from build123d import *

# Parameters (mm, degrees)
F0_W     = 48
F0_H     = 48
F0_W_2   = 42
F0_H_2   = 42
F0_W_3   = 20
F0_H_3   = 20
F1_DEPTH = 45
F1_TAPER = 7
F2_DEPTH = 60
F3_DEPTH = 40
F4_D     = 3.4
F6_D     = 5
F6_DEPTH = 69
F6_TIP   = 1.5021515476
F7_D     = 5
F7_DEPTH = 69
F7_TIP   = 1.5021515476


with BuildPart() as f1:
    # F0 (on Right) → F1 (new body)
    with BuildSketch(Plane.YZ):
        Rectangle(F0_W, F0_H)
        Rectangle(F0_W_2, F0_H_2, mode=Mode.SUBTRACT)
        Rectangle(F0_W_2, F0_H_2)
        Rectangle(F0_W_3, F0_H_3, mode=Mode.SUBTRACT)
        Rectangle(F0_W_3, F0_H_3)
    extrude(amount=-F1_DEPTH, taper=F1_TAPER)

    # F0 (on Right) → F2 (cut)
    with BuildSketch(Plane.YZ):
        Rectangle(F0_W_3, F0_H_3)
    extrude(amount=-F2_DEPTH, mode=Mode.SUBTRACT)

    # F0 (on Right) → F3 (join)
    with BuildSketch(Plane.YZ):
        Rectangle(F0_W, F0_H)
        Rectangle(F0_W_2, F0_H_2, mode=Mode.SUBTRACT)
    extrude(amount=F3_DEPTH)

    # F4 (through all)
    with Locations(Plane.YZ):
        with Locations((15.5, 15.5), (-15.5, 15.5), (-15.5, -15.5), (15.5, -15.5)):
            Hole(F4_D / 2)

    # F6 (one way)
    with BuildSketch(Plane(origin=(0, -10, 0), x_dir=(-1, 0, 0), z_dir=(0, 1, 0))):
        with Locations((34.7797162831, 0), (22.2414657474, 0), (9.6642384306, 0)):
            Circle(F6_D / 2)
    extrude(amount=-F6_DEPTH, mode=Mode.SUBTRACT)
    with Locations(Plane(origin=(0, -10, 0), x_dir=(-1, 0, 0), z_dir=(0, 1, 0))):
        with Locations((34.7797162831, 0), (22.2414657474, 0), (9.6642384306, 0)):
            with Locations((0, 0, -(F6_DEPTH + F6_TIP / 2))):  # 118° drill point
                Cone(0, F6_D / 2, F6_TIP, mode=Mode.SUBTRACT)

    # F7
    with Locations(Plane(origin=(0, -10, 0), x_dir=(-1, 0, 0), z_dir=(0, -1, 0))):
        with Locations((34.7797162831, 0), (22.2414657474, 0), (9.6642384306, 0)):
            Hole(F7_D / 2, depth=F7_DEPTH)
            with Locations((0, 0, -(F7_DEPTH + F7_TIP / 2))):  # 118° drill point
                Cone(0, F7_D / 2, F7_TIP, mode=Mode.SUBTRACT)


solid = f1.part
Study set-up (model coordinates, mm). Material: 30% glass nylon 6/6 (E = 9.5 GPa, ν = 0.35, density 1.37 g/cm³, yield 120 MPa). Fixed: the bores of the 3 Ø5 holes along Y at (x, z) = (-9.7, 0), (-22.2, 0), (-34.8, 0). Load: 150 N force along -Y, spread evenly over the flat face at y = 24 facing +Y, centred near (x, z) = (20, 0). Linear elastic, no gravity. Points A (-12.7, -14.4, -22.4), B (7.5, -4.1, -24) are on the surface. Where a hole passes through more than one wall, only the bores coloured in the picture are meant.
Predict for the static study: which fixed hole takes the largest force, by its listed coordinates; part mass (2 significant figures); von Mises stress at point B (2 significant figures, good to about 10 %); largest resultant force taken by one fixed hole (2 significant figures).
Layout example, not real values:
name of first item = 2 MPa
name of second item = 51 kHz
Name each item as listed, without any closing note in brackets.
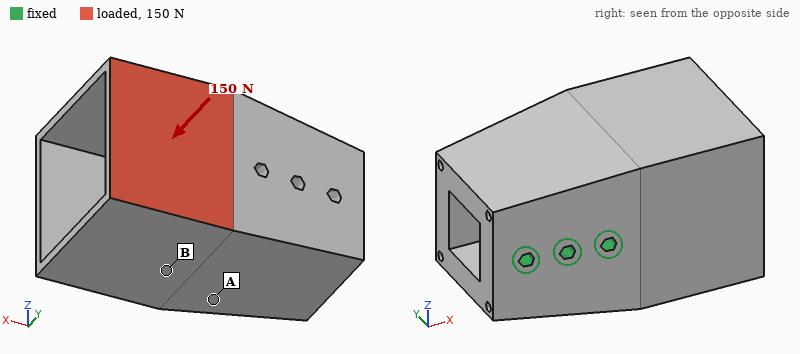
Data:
which fixed hole takes the largest force, by its listed coordinates = (-9.7, 0)
part mass = 110 g
von Mises stress at point B = 1.3 MPa
largest resultant force taken by one fixed hole = 240 N
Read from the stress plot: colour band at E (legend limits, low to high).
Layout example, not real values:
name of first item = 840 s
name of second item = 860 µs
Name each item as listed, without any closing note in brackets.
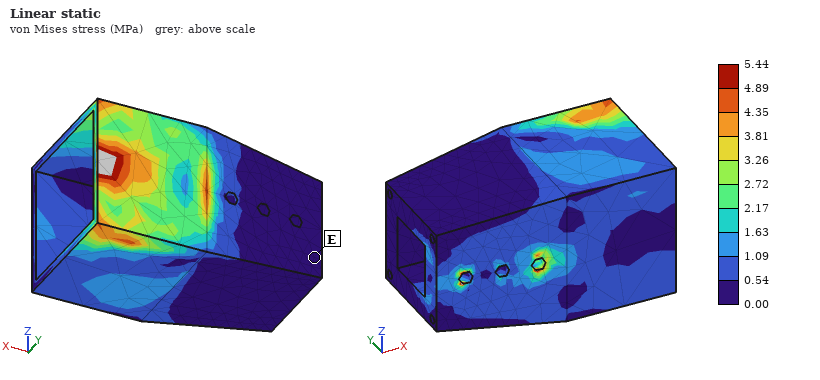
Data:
colour band at E = 0.00 to 0.54 MPa
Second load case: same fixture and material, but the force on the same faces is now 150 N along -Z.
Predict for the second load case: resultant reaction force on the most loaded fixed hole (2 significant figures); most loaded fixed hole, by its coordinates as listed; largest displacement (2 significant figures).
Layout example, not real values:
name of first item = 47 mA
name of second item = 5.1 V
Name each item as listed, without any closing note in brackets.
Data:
resultant reaction force on the most loaded fixed hole = 280 N
most loaded fixed hole, by its coordinates as listed = (-9.7, 0)
largest displacement = 66 µm
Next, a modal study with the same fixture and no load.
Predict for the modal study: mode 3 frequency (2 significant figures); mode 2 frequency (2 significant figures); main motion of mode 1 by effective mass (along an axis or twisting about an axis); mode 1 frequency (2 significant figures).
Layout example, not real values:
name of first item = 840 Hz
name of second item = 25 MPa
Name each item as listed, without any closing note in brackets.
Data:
mode 3 frequency = 2500 Hz
mode 2 frequency = 2000 Hz
main motion of mode 1 by effective mass = along Z
mode 1 frequency = 1700 Hz
